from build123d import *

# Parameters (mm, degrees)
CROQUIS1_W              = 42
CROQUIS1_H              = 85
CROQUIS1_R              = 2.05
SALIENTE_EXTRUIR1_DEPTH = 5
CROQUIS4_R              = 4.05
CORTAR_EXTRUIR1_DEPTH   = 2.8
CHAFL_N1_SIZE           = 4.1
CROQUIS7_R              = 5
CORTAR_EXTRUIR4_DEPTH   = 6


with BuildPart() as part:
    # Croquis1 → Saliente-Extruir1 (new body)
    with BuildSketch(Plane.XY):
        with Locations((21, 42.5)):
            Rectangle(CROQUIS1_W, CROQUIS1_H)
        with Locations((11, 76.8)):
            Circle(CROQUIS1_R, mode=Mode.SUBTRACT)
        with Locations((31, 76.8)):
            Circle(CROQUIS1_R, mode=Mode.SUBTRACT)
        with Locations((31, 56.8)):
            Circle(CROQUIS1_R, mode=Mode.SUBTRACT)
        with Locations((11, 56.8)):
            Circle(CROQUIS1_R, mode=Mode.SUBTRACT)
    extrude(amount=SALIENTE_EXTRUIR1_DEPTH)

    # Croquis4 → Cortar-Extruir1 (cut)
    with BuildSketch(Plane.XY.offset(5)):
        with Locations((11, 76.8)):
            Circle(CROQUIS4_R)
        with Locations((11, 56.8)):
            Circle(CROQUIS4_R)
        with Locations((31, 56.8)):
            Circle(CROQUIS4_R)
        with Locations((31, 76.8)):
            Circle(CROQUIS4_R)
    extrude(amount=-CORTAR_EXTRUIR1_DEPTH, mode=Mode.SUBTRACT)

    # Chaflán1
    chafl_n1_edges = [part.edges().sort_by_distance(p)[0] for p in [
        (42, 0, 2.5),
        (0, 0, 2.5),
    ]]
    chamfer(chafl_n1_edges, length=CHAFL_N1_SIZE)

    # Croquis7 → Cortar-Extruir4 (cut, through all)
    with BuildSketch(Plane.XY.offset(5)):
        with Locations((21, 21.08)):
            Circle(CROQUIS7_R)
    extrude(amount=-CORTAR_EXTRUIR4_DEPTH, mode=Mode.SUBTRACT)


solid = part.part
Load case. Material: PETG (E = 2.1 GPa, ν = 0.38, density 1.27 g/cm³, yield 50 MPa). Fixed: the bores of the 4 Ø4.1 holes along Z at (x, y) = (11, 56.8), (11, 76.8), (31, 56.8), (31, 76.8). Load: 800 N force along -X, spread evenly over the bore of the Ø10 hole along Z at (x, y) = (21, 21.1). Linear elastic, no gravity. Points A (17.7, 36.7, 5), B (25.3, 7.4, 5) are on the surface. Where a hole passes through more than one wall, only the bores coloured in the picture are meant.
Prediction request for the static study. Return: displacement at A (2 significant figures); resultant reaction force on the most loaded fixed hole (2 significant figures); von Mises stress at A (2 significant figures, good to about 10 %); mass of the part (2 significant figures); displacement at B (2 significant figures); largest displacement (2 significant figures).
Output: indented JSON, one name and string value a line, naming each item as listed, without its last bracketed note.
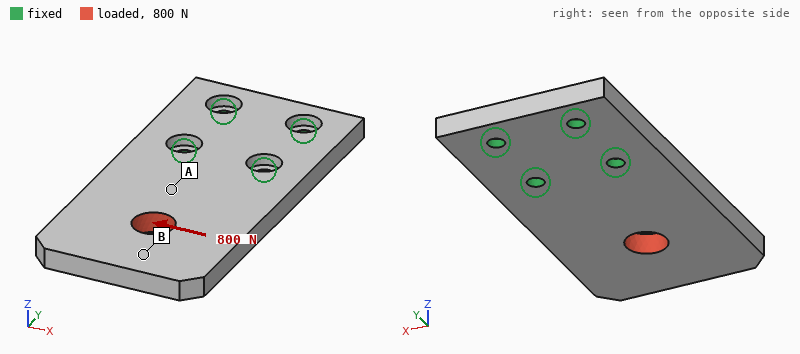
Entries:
{
  "displacement at A": "0.31 mm",
  "resultant reaction force on the most loaded fixed hole": "920 N",
  "von Mises stress at A": "10 MPa",
  "mass of the part": "21 g",
  "displacement at B": "0.81 mm",
  "largest displacement": "0.97 mm"
}
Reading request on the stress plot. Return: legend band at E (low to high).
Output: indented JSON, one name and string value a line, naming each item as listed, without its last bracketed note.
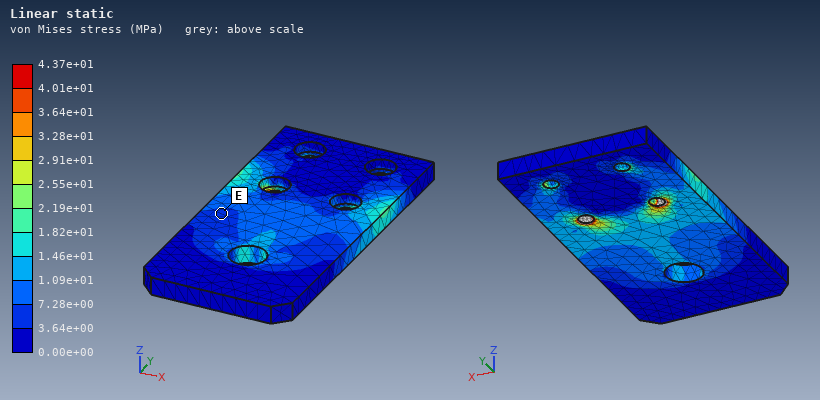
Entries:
{
  "legend band at E": "3.64e+00 to 7.28e+00 MPa"
}
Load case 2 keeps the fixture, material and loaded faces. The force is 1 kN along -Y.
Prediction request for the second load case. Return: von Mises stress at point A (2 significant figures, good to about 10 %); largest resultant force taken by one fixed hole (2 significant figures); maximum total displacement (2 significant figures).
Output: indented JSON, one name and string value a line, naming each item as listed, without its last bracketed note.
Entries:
{
  "von Mises stress at point A": "6.3 MPa",
  "largest resultant force taken by one fixed hole": "360 N",
  "maximum total displacement": "0.53 mm"
}
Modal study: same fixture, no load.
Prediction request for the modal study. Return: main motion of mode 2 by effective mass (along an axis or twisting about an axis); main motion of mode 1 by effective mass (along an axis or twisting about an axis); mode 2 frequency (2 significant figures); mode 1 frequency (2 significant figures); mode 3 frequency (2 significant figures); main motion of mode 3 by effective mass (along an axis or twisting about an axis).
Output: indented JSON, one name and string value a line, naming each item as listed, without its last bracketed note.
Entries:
{
  "main motion of mode 2 by effective mass": "twisting about Y",
  "main motion of mode 1 by effective mass": "along Z",
  "mode 2 frequency": "860 Hz",
  "mode 1 frequency": "290 Hz",
  "mode 3 frequency": "1600 Hz",
  "main motion of mode 3 by effective mass": "along X"
}
